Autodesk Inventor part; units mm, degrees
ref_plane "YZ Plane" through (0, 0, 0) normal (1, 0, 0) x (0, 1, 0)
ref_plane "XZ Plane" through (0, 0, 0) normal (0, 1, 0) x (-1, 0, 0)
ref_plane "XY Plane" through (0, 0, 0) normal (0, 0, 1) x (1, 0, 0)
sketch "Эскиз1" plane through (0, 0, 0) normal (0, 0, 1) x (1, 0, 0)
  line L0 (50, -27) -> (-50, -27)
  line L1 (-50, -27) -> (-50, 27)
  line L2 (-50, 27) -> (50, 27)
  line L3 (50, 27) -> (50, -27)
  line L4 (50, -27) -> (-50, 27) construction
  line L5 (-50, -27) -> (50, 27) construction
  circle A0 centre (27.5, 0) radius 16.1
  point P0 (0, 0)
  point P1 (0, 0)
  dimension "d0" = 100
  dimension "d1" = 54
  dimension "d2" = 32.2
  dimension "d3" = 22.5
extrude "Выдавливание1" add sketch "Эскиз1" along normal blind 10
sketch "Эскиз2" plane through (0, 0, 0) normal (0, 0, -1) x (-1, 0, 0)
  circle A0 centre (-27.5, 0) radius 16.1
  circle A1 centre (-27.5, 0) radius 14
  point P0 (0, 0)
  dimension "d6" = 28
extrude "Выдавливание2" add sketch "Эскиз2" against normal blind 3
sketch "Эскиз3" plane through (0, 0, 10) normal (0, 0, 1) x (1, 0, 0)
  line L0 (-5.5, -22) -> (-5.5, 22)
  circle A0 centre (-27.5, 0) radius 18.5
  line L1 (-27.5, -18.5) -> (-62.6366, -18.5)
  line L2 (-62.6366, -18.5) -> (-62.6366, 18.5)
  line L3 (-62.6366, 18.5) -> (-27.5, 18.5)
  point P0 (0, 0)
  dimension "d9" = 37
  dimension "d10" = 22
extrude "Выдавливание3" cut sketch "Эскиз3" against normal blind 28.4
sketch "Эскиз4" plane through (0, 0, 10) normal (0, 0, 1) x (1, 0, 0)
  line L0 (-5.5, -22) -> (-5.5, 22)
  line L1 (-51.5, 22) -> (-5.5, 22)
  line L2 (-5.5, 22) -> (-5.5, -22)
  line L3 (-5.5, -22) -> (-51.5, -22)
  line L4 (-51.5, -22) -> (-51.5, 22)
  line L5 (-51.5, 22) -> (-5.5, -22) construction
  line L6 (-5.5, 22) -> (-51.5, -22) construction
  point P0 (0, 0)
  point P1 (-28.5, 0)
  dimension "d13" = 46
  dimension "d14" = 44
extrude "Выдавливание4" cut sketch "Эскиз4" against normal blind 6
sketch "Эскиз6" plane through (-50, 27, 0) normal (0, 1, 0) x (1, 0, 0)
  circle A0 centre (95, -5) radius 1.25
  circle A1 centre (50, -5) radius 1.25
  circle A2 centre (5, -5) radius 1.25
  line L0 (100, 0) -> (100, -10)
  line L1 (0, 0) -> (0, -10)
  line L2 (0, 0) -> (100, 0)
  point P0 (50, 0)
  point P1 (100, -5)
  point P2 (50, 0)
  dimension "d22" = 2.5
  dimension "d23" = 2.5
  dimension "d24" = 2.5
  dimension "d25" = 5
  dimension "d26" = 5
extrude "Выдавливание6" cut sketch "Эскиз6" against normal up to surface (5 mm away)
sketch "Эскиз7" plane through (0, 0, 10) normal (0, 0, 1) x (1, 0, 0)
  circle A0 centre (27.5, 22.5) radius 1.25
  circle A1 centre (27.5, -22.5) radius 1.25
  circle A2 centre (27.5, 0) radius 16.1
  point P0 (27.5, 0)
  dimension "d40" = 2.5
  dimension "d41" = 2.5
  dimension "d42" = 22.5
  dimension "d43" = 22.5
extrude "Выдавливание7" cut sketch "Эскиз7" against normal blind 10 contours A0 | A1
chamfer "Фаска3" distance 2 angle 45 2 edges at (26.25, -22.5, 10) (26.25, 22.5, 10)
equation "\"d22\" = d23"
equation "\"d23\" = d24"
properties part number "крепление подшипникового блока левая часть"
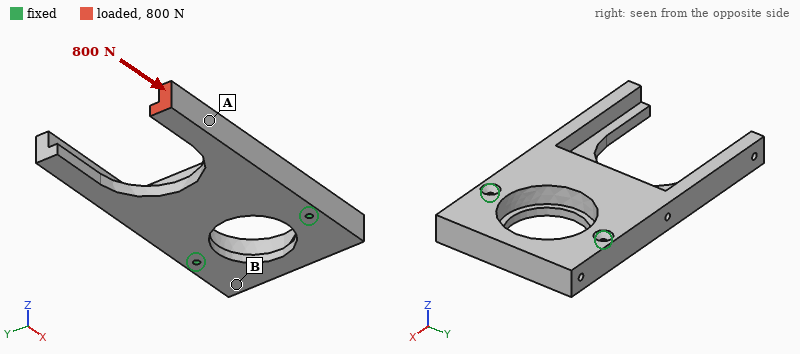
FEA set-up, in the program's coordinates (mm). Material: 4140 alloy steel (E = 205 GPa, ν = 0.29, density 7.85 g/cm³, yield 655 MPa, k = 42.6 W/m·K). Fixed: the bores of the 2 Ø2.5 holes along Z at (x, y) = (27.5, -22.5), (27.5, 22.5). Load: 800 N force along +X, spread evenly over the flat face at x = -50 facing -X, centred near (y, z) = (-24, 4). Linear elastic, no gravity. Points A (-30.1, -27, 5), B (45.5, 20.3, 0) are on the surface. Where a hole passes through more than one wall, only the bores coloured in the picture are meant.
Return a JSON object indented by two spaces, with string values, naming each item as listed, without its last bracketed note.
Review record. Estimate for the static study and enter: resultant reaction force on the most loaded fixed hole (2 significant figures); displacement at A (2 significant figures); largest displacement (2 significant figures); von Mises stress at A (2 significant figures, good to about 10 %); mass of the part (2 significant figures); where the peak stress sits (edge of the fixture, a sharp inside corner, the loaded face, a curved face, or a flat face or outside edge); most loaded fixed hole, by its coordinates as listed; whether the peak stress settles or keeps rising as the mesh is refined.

{
  "resultant reaction force on the most loaded fixed hole": "820 N",
  "displacement at A": "5.2 µm",
  "largest displacement": "8.4 µm",
  "von Mises stress at A": "13 MPa",
  "mass of the part": "230 g",
  "where the peak stress sits": "edge of the fixture",
  "most loaded fixed hole, by its coordinates as listed": "(27.5, -22.5)",
  "whether the peak stress settles or keeps rising as the mesh is refined": "keeps rising"
}
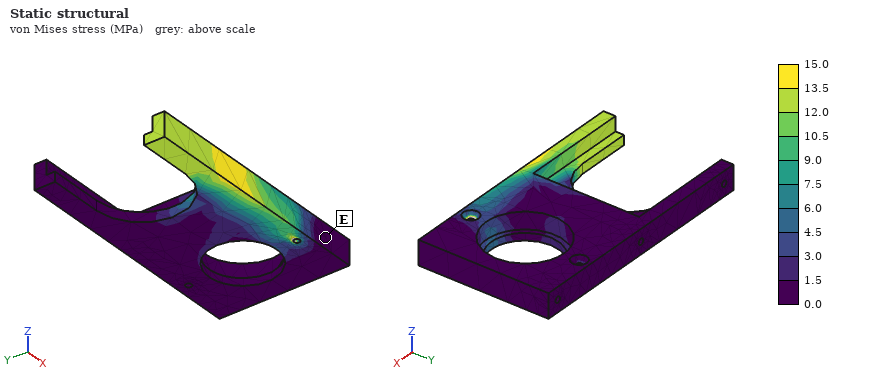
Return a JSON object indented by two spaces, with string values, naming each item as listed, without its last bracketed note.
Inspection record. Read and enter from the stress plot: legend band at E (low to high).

{
  "legend band at E": "0.0 to 1.5 MPa"
}
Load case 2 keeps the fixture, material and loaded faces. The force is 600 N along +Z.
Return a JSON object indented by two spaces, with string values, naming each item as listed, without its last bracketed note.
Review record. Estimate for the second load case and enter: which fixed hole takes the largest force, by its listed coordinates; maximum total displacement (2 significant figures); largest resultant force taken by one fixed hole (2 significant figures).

{
  "which fixed hole takes the largest force, by its listed coordinates": "(27.5, -22.5)",
  "maximum total displacement": "0.47 mm",
  "largest resultant force taken by one fixed hole": "550 N"
}
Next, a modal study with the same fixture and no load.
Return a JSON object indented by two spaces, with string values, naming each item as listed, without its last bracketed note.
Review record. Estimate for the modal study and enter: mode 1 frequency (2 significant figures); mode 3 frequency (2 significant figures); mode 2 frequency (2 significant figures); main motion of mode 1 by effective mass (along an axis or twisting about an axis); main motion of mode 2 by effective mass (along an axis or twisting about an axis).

{
  "mode 1 frequency": "1600 Hz",
  "mode 3 frequency": "4000 Hz",
  "mode 2 frequency": "2400 Hz",
  "main motion of mode 1 by effective mass": "along Z",
  "main motion of mode 2 by effective mass": "twisting about X"
}
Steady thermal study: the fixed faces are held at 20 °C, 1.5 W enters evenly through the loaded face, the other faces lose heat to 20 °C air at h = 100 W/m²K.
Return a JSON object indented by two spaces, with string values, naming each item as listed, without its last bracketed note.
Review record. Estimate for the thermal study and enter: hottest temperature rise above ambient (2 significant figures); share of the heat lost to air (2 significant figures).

{
  "hottest temperature rise above ambient": "14 K",
  "share of the heat lost to air": "85 %"
}
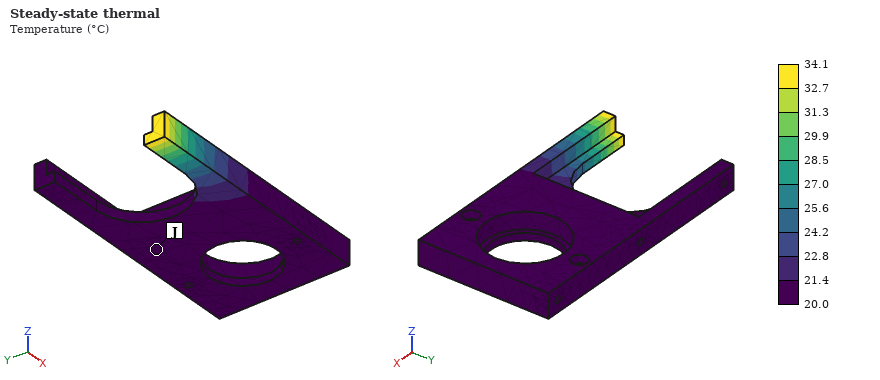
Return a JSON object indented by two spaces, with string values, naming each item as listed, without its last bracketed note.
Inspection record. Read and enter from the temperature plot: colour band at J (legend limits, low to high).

{
  "colour band at J": "20.0 to 21.4 °C"
}
